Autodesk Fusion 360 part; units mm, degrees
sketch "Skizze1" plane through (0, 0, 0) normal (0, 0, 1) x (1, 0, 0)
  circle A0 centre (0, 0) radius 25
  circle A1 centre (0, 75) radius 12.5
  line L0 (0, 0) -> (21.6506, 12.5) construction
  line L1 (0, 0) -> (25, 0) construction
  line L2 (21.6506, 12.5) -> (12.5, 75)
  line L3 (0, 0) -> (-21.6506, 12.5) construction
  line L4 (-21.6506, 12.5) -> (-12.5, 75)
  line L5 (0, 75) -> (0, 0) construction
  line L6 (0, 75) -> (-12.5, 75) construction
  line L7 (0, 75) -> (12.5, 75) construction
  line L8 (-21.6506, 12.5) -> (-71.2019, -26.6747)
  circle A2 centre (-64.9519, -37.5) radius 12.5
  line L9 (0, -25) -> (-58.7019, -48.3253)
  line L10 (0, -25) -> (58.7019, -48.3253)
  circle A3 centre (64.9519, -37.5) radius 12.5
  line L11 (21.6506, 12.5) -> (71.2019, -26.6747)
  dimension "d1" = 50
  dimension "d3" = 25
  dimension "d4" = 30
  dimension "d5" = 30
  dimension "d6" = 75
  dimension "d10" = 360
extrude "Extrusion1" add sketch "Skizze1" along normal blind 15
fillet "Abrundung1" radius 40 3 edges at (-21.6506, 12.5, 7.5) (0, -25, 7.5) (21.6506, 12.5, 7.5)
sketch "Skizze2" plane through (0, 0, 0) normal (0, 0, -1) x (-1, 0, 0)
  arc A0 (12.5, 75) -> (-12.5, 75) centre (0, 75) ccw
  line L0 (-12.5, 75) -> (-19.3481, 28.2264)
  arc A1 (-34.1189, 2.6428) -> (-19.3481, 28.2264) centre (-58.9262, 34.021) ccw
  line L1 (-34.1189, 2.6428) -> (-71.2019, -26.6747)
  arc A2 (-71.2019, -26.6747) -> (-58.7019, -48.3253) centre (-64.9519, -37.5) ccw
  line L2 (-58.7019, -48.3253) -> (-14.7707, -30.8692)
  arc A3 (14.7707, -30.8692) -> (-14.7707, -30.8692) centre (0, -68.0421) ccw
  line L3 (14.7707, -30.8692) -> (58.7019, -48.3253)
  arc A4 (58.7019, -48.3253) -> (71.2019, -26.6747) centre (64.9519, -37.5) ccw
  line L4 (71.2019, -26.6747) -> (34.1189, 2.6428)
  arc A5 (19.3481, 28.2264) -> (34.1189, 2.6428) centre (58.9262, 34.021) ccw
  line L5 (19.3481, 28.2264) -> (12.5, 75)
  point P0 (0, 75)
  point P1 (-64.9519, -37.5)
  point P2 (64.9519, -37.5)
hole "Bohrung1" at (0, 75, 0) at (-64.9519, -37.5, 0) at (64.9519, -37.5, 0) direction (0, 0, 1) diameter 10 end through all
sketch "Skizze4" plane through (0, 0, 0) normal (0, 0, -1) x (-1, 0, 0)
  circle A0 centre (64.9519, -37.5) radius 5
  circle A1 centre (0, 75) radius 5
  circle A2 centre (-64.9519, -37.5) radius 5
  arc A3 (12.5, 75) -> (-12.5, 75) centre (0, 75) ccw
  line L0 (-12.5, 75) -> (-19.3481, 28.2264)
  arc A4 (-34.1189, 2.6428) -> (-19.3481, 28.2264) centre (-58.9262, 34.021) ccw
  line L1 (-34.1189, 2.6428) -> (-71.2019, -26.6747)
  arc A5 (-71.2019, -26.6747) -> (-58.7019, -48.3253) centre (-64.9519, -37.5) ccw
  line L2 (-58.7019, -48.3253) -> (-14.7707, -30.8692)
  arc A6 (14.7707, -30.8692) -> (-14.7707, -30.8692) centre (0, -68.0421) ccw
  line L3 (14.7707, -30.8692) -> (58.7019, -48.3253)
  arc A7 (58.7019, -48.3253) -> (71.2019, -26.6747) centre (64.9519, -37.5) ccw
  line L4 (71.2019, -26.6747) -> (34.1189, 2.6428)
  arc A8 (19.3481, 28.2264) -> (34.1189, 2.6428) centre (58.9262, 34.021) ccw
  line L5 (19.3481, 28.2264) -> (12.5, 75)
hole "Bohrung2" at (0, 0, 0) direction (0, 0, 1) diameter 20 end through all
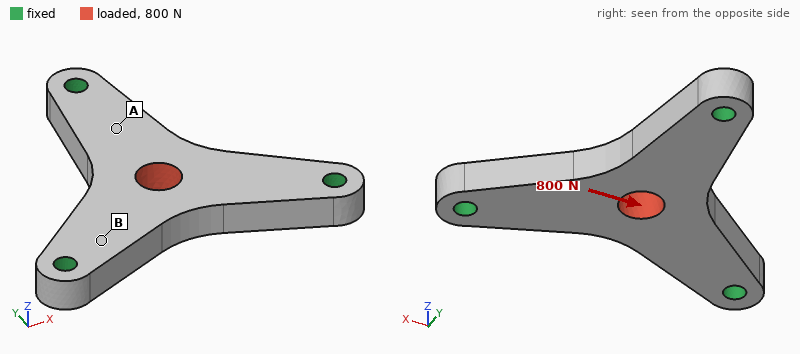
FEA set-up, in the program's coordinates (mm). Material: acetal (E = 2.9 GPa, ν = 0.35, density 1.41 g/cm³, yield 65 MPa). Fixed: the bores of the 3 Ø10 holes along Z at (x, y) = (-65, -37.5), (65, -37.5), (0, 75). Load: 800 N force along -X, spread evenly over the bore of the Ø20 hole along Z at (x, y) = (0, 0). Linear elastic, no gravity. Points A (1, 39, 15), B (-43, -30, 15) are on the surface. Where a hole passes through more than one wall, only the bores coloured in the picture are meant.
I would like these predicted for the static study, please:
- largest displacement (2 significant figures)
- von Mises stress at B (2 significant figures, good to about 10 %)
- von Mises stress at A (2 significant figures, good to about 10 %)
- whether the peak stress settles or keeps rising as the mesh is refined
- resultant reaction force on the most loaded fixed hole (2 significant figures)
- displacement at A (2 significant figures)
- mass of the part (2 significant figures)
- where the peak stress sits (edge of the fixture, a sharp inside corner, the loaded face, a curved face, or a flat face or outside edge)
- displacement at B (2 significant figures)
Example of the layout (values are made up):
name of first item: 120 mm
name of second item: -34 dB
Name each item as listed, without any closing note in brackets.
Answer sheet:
largest displacement: 36 µm
von Mises stress at B: 0.95 MPa
von Mises stress at A: 0.21 MPa
whether the peak stress settles or keeps rising as the mesh is refined: keeps rising
resultant reaction force on the most loaded fixed hole: 420 N
displacement at A: 18 µm
mass of the part: 160 g
where the peak stress sits: edge of the fixture
displacement at B: 8.3 µm
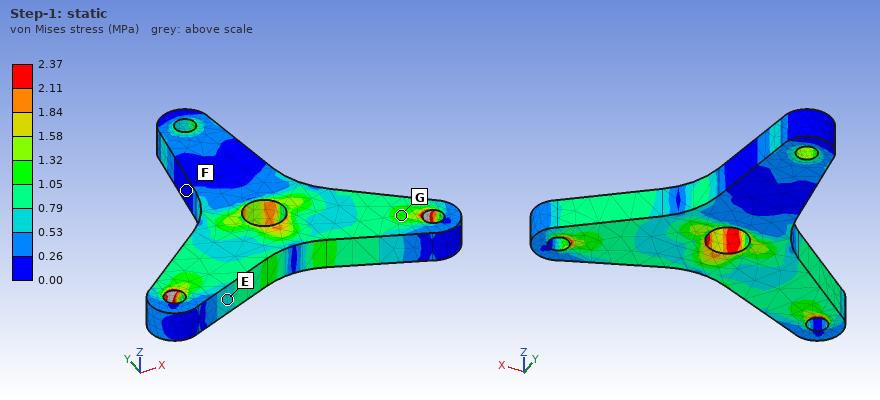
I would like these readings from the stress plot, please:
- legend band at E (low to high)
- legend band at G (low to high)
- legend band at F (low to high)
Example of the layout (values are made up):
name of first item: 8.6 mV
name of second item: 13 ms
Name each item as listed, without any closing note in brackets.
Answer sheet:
legend band at E: 0.53 to 0.79 MPa
legend band at G: 1.05 to 1.32 MPa
legend band at F: 0.00 to 0.26 MPa
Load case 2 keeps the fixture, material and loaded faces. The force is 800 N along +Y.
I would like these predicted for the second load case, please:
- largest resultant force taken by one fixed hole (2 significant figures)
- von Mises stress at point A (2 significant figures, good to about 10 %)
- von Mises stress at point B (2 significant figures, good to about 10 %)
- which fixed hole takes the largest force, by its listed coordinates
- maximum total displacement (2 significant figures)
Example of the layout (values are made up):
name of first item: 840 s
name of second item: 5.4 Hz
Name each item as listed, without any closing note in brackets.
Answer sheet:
largest resultant force taken by one fixed hole: 490 N
von Mises stress at point A: 0.87 MPa
von Mises stress at point B: 0.62 MPa
which fixed hole takes the largest force, by its listed coordinates: (0, 75)
maximum total displacement: 38 µm
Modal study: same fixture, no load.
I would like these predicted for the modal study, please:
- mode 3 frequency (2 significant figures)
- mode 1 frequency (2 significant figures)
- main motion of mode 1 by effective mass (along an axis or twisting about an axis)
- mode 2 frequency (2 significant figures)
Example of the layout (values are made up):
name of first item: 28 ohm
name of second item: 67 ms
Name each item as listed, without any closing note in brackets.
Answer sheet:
mode 3 frequency: 2200 Hz
mode 1 frequency: 1100 Hz
main motion of mode 1 by effective mass: along Z
mode 2 frequency: 2200 Hz
